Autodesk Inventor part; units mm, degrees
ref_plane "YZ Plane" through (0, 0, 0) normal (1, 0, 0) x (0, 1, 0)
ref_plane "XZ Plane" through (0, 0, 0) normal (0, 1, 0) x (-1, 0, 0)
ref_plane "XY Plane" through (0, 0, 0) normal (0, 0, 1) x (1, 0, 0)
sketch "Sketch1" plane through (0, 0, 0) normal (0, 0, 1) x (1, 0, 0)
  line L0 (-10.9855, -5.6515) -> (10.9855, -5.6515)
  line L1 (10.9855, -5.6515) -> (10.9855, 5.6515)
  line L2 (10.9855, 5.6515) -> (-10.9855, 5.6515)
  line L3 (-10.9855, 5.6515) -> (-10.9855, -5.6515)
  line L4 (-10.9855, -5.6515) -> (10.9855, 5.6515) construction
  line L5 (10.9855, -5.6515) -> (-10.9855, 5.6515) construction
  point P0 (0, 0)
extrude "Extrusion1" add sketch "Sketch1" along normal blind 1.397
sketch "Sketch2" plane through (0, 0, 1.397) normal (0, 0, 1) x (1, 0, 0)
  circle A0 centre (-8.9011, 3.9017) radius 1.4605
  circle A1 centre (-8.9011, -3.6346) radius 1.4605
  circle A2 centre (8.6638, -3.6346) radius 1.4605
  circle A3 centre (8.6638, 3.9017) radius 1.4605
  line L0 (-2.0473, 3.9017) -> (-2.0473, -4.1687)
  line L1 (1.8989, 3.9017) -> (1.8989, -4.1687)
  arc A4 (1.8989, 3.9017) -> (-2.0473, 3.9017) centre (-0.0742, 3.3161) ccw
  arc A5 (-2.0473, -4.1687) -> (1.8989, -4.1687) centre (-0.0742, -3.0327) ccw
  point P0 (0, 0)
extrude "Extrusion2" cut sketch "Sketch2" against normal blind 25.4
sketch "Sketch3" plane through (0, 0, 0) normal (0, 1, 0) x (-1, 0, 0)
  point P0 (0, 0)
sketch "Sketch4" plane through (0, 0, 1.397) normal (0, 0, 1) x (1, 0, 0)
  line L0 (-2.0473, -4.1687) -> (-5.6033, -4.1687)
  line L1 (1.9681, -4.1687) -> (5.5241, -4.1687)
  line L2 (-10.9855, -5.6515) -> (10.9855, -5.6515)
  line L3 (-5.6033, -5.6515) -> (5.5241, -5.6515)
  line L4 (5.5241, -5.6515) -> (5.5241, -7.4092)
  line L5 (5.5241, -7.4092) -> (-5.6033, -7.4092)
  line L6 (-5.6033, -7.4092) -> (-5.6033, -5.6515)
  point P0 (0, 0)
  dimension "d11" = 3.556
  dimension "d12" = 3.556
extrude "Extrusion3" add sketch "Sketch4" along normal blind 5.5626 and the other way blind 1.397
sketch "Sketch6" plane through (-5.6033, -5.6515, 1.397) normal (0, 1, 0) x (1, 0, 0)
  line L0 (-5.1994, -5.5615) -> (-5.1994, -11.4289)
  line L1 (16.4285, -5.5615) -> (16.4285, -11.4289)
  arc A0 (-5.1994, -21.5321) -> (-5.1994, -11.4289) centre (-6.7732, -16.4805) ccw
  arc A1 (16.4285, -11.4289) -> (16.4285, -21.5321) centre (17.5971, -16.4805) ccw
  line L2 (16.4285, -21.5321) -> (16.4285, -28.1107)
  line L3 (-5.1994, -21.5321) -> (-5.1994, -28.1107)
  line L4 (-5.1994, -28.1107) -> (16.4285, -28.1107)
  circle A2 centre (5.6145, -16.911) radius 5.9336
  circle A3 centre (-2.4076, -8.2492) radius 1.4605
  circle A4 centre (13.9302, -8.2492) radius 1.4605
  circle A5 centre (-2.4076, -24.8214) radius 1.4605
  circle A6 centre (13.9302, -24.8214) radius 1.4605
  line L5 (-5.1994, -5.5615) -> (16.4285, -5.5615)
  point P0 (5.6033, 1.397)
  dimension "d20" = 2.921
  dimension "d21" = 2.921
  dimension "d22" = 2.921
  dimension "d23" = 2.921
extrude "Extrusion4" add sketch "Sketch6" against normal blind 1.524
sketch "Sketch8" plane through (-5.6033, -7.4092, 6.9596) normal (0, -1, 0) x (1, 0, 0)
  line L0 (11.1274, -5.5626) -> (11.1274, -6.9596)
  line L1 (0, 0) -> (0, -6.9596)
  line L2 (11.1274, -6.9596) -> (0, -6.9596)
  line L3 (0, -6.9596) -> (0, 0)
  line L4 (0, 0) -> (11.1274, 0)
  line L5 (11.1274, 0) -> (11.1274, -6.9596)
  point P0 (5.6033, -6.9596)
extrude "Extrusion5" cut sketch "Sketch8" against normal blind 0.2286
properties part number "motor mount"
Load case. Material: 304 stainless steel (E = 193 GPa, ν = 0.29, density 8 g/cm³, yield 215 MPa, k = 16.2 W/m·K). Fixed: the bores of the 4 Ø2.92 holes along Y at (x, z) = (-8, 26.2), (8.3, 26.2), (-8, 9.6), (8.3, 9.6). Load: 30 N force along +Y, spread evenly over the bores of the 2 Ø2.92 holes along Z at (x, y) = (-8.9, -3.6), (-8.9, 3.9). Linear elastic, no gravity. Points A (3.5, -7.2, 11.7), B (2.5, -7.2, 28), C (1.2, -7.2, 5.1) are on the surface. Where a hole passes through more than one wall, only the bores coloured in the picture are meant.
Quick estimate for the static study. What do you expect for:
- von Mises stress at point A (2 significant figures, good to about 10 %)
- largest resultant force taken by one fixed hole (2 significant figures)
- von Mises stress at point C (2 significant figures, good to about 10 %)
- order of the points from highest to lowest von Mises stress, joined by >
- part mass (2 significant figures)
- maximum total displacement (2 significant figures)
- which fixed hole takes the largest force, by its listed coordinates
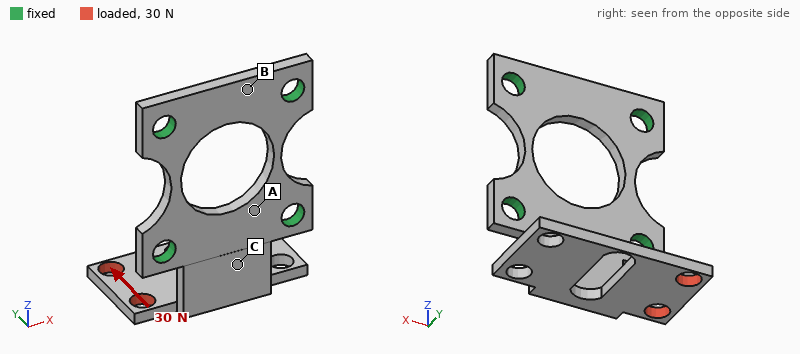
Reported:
17 MPa
40 N
41 MPa
C > A > B
6.5 g
49 µm
(-8, 9.6)
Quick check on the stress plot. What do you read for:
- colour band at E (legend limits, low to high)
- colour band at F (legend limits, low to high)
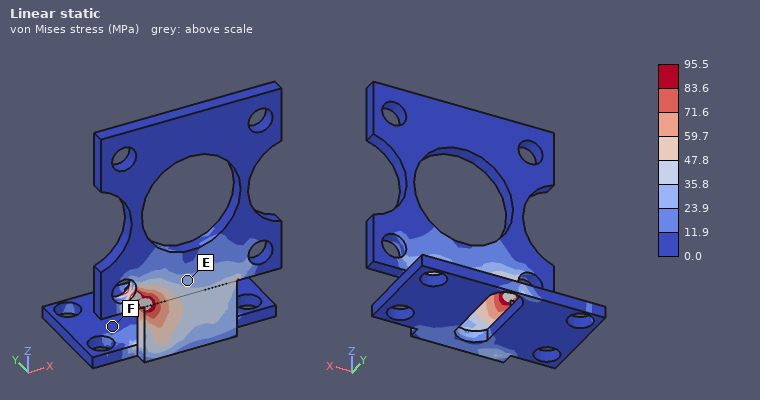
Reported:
23.9 to 35.8 MPa
0.0 to 11.9 MPa
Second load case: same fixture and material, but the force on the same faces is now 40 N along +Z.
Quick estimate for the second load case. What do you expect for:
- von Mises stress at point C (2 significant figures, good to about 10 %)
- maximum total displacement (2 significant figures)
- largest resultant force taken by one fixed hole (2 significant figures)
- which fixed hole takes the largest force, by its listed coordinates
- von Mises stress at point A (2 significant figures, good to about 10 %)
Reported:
55 MPa
0.12 mm
44 N
(-8, 9.6)
20 MPa
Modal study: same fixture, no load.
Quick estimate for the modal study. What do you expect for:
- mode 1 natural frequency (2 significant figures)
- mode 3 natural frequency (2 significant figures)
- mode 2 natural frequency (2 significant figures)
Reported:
2900 Hz
7300 Hz
4600 Hz
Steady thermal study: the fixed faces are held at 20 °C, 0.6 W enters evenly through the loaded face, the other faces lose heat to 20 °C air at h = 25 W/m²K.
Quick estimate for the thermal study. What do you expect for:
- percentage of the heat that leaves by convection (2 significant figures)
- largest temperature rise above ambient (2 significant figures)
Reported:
50 %
47 K
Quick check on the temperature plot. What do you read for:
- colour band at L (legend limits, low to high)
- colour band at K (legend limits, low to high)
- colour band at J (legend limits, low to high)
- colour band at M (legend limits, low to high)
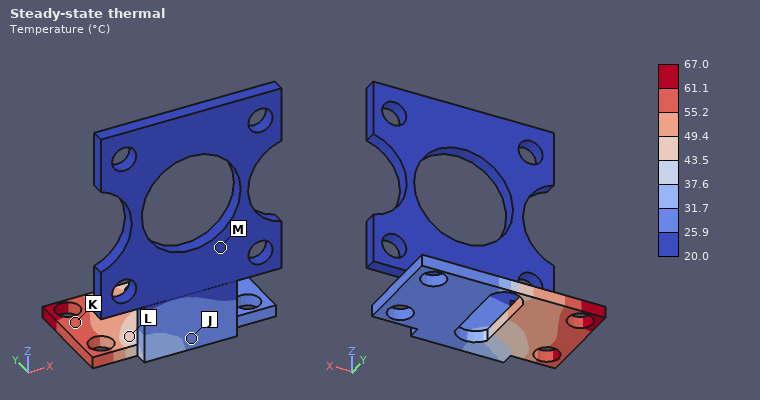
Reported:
43.5 to 49.4 °C
55.2 to 61.1 °C
25.9 to 31.7 °C
20.0 to 25.9 °C
